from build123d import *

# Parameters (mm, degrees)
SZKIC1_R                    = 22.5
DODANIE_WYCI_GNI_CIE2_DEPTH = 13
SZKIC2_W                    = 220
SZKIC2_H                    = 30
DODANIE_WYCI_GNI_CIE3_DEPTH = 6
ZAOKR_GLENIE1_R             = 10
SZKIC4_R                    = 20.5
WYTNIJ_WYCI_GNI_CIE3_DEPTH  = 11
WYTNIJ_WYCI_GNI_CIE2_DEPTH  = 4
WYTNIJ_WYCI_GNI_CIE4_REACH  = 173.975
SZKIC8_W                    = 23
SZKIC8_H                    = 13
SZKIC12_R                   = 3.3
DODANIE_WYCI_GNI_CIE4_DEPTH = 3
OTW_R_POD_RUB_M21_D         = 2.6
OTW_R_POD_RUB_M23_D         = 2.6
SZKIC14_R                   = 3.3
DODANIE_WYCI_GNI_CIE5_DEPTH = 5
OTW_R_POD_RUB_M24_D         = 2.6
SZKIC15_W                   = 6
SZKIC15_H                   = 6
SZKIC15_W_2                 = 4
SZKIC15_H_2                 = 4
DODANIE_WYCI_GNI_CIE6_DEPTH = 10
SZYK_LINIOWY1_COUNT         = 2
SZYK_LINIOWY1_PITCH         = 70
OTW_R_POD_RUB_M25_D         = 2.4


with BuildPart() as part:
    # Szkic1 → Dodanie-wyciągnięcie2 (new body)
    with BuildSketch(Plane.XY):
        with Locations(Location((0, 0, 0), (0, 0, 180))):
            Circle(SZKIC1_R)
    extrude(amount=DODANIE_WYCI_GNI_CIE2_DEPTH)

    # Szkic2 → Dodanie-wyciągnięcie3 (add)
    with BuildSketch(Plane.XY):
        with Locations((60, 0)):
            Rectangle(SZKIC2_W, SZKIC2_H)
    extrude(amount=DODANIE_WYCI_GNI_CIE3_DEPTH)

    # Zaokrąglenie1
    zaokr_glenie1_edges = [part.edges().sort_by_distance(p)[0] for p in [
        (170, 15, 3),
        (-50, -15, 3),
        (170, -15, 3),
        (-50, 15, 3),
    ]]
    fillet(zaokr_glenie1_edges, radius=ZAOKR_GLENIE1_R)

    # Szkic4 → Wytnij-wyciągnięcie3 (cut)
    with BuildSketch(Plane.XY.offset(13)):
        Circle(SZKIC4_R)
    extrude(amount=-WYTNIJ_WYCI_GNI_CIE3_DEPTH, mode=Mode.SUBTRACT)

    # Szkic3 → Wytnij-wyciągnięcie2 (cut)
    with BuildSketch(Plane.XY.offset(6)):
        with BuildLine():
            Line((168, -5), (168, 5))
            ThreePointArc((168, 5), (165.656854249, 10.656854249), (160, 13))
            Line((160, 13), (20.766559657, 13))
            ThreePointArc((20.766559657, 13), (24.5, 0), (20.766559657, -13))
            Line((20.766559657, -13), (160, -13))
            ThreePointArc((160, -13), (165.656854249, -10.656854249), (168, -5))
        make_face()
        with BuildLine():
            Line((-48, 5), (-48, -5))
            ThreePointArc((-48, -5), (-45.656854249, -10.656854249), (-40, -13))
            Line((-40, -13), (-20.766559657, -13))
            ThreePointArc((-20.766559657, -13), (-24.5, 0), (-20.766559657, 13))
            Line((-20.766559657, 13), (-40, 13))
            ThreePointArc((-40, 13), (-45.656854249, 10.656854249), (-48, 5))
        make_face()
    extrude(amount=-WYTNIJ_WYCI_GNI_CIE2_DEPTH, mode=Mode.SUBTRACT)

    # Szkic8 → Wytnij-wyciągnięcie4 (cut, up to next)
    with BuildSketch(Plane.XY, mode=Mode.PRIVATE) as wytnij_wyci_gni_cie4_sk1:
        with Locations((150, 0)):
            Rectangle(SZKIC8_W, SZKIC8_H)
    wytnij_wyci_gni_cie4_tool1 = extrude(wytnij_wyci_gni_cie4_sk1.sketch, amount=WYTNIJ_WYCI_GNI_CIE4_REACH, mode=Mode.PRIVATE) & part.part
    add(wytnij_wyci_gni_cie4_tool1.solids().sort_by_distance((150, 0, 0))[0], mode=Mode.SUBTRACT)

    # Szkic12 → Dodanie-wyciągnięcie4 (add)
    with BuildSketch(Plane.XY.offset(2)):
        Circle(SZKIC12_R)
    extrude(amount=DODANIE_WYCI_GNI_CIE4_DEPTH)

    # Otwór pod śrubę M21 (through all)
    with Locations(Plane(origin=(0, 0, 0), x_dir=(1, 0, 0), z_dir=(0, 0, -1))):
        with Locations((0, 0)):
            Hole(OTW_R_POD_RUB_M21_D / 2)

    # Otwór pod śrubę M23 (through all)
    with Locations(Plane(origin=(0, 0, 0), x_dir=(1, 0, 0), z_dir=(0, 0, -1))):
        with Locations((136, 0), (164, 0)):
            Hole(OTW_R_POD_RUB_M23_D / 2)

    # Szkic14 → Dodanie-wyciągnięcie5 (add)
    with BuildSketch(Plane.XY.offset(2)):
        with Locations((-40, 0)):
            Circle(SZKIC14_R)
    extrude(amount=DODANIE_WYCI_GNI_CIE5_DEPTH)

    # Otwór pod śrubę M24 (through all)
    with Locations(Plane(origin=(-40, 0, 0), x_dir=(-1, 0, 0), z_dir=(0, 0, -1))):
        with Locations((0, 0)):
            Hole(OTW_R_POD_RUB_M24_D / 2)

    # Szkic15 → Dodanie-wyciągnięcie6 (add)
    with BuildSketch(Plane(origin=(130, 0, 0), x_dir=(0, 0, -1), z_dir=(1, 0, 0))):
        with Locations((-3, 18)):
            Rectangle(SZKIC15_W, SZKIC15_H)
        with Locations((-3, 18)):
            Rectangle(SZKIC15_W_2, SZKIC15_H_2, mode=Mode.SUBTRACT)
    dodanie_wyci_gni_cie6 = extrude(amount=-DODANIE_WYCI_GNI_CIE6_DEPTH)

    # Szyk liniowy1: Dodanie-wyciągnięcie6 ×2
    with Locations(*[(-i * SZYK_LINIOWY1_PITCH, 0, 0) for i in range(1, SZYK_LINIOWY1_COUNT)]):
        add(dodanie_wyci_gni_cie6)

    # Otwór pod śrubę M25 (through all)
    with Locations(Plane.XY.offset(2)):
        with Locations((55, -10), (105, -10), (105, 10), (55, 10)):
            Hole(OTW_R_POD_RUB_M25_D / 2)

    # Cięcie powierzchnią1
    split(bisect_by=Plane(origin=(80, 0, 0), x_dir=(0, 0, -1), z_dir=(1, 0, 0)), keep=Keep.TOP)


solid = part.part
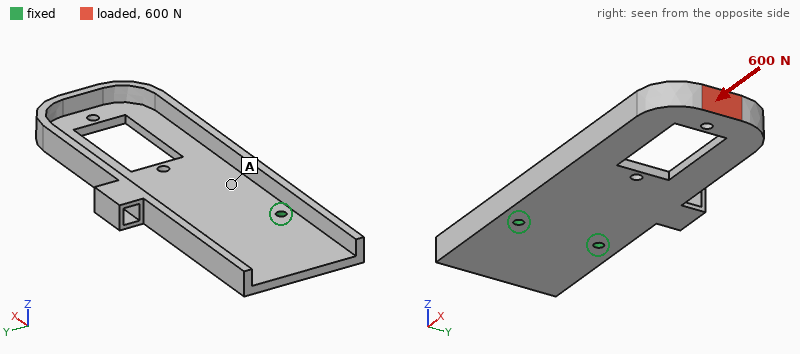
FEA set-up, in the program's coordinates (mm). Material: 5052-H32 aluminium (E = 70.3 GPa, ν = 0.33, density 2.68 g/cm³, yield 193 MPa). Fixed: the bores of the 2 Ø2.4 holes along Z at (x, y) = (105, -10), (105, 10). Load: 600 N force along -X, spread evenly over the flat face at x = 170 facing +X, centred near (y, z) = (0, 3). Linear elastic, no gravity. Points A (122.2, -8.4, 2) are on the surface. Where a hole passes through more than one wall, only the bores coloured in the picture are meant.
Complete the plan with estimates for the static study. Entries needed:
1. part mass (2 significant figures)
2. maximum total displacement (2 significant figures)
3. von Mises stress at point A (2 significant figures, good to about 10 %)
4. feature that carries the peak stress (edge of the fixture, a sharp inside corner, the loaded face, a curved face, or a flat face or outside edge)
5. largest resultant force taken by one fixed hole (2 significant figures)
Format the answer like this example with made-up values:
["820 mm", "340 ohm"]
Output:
["17 g", "0.29 mm", "8.8 MPa", "a curved face", "300 N"]
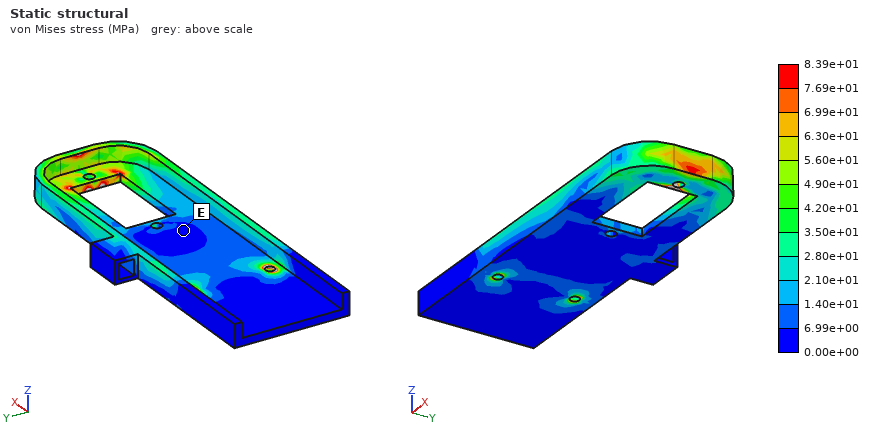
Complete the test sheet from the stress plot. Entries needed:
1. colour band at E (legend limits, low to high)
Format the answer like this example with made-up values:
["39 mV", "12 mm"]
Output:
["0.00e+00 to 6.99e+00 MPa"]
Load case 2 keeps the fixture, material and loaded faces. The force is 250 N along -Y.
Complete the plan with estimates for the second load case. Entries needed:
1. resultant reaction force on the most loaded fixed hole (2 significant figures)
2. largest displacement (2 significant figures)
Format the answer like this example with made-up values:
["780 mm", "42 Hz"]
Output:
["790 N", "0.23 mm"]
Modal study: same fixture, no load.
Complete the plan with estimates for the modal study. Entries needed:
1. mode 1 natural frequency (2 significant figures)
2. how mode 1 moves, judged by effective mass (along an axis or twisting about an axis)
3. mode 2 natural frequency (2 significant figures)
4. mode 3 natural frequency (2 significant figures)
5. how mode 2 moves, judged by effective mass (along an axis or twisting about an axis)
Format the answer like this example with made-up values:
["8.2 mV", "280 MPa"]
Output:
["760 Hz", "along Z", "1900 Hz", "3800 Hz", "twisting about X"]
